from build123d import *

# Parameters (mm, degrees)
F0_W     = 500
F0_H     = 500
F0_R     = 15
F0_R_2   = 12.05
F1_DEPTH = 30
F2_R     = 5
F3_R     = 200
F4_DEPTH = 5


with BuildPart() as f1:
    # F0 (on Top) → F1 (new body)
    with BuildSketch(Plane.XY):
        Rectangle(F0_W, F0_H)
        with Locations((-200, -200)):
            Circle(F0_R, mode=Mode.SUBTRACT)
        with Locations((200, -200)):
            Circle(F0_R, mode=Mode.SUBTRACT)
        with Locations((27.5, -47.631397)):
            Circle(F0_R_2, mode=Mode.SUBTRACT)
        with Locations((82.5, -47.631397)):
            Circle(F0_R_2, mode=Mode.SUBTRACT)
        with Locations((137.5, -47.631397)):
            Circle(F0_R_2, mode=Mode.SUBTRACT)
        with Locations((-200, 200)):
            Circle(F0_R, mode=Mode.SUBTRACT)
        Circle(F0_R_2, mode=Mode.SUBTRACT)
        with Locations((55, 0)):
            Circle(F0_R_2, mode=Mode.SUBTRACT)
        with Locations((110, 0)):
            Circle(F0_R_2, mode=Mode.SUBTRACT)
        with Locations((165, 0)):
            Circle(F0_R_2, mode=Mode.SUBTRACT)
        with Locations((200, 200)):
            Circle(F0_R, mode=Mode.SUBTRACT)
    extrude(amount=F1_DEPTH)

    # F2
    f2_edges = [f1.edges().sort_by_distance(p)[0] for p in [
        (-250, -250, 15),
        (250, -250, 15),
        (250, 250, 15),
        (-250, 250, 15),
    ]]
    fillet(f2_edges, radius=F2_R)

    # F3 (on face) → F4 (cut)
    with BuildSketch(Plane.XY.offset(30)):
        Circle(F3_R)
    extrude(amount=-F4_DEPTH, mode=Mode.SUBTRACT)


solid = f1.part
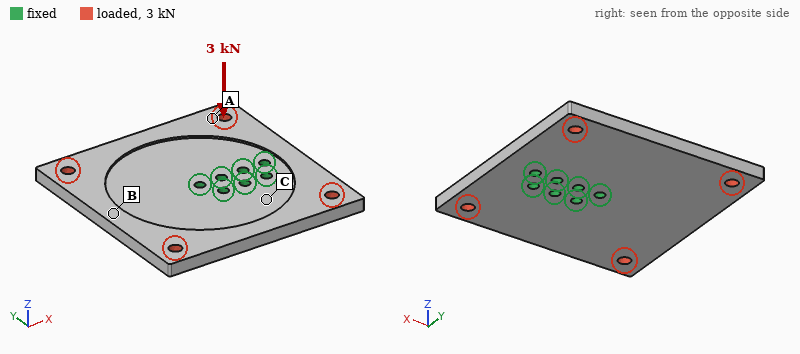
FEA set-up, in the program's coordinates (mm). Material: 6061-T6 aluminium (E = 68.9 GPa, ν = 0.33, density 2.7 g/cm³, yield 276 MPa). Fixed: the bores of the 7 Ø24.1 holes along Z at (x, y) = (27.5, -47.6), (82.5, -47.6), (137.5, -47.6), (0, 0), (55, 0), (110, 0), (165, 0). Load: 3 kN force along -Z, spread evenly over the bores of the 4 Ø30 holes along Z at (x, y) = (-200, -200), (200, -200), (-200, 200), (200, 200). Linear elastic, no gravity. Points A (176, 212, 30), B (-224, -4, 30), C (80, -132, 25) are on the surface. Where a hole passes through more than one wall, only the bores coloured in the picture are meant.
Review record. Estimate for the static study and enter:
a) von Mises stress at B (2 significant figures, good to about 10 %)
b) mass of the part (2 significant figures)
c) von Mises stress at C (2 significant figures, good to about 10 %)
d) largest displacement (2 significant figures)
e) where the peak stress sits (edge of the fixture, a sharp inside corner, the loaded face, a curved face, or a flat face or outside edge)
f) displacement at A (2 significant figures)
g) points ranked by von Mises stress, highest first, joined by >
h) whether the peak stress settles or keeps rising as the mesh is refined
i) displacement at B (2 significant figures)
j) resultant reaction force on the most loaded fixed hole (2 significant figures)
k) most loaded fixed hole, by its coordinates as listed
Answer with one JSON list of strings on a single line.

["3.9 MPa", "18 kg", "2.0 MPa", "0.22 mm", "edge of the fixture", "0.070 mm", "B > C > A", "keeps rising", "0.11 mm", "2.2 kN", "(0, 0)"]
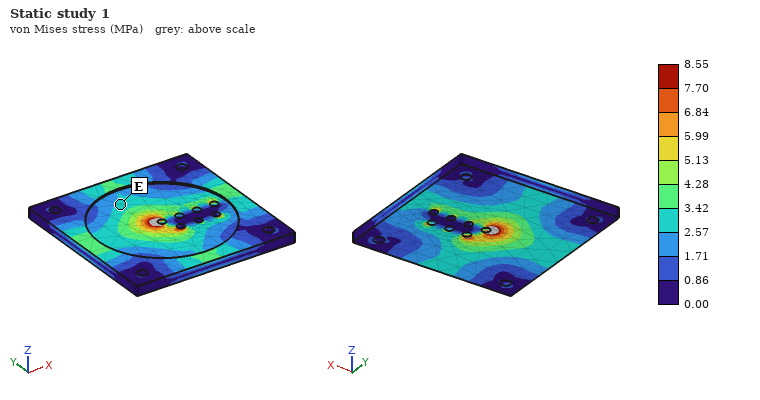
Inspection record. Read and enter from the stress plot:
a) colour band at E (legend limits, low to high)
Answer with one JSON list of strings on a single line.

["2.57 to 3.42 MPa"]
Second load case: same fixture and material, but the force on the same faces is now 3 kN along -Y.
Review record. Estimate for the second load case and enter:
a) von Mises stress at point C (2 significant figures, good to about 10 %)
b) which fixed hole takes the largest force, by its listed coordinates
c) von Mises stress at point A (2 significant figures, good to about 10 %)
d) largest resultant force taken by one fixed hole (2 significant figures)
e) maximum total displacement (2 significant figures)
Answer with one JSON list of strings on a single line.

["0.28 MPa", "(0, 0)", "0.22 MPa", "1.7 kN", "5.8 µm"]
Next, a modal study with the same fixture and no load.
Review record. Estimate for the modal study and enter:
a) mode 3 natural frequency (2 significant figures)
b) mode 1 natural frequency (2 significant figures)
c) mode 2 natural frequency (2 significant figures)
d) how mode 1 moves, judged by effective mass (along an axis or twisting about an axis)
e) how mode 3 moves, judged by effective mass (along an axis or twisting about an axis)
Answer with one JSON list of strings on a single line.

["410 Hz", "240 Hz", "260 Hz", "along Z", "along Z"]
